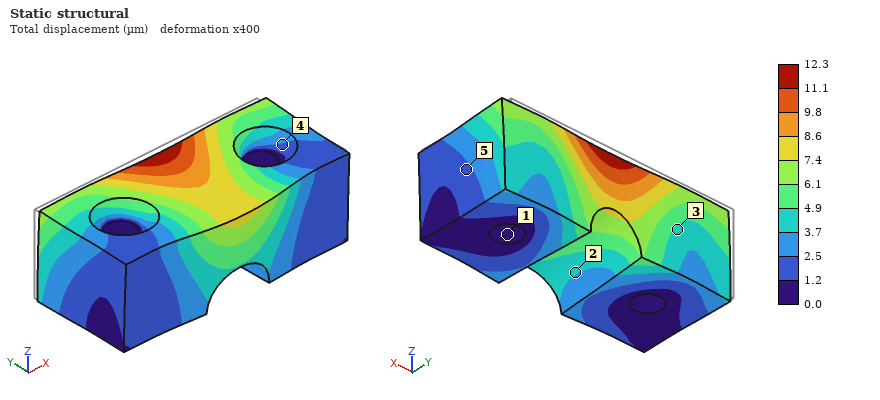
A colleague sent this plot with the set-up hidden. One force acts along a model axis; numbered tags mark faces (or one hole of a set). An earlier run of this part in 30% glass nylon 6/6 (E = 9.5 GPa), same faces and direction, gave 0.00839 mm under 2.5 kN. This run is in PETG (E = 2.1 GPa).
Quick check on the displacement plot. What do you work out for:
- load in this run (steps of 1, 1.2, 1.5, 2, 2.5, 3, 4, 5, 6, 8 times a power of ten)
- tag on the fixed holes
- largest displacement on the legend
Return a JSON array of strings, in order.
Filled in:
["800 N", "1", "12.3 µm"]
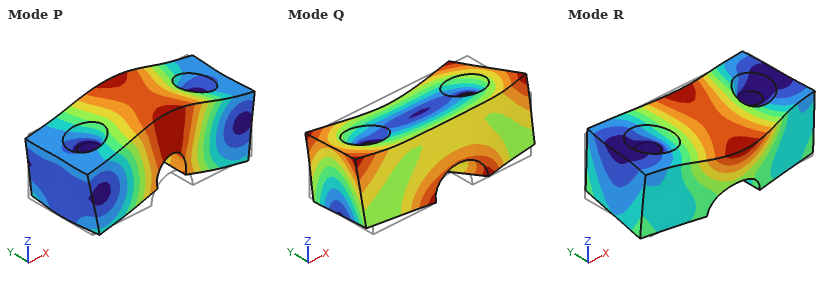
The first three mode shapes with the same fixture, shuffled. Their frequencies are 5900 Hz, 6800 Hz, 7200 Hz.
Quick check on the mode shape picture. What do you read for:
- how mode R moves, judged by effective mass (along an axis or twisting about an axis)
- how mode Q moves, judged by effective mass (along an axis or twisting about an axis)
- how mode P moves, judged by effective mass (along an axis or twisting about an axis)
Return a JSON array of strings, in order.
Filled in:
["along Y", "twisting about X", "along Z"]
